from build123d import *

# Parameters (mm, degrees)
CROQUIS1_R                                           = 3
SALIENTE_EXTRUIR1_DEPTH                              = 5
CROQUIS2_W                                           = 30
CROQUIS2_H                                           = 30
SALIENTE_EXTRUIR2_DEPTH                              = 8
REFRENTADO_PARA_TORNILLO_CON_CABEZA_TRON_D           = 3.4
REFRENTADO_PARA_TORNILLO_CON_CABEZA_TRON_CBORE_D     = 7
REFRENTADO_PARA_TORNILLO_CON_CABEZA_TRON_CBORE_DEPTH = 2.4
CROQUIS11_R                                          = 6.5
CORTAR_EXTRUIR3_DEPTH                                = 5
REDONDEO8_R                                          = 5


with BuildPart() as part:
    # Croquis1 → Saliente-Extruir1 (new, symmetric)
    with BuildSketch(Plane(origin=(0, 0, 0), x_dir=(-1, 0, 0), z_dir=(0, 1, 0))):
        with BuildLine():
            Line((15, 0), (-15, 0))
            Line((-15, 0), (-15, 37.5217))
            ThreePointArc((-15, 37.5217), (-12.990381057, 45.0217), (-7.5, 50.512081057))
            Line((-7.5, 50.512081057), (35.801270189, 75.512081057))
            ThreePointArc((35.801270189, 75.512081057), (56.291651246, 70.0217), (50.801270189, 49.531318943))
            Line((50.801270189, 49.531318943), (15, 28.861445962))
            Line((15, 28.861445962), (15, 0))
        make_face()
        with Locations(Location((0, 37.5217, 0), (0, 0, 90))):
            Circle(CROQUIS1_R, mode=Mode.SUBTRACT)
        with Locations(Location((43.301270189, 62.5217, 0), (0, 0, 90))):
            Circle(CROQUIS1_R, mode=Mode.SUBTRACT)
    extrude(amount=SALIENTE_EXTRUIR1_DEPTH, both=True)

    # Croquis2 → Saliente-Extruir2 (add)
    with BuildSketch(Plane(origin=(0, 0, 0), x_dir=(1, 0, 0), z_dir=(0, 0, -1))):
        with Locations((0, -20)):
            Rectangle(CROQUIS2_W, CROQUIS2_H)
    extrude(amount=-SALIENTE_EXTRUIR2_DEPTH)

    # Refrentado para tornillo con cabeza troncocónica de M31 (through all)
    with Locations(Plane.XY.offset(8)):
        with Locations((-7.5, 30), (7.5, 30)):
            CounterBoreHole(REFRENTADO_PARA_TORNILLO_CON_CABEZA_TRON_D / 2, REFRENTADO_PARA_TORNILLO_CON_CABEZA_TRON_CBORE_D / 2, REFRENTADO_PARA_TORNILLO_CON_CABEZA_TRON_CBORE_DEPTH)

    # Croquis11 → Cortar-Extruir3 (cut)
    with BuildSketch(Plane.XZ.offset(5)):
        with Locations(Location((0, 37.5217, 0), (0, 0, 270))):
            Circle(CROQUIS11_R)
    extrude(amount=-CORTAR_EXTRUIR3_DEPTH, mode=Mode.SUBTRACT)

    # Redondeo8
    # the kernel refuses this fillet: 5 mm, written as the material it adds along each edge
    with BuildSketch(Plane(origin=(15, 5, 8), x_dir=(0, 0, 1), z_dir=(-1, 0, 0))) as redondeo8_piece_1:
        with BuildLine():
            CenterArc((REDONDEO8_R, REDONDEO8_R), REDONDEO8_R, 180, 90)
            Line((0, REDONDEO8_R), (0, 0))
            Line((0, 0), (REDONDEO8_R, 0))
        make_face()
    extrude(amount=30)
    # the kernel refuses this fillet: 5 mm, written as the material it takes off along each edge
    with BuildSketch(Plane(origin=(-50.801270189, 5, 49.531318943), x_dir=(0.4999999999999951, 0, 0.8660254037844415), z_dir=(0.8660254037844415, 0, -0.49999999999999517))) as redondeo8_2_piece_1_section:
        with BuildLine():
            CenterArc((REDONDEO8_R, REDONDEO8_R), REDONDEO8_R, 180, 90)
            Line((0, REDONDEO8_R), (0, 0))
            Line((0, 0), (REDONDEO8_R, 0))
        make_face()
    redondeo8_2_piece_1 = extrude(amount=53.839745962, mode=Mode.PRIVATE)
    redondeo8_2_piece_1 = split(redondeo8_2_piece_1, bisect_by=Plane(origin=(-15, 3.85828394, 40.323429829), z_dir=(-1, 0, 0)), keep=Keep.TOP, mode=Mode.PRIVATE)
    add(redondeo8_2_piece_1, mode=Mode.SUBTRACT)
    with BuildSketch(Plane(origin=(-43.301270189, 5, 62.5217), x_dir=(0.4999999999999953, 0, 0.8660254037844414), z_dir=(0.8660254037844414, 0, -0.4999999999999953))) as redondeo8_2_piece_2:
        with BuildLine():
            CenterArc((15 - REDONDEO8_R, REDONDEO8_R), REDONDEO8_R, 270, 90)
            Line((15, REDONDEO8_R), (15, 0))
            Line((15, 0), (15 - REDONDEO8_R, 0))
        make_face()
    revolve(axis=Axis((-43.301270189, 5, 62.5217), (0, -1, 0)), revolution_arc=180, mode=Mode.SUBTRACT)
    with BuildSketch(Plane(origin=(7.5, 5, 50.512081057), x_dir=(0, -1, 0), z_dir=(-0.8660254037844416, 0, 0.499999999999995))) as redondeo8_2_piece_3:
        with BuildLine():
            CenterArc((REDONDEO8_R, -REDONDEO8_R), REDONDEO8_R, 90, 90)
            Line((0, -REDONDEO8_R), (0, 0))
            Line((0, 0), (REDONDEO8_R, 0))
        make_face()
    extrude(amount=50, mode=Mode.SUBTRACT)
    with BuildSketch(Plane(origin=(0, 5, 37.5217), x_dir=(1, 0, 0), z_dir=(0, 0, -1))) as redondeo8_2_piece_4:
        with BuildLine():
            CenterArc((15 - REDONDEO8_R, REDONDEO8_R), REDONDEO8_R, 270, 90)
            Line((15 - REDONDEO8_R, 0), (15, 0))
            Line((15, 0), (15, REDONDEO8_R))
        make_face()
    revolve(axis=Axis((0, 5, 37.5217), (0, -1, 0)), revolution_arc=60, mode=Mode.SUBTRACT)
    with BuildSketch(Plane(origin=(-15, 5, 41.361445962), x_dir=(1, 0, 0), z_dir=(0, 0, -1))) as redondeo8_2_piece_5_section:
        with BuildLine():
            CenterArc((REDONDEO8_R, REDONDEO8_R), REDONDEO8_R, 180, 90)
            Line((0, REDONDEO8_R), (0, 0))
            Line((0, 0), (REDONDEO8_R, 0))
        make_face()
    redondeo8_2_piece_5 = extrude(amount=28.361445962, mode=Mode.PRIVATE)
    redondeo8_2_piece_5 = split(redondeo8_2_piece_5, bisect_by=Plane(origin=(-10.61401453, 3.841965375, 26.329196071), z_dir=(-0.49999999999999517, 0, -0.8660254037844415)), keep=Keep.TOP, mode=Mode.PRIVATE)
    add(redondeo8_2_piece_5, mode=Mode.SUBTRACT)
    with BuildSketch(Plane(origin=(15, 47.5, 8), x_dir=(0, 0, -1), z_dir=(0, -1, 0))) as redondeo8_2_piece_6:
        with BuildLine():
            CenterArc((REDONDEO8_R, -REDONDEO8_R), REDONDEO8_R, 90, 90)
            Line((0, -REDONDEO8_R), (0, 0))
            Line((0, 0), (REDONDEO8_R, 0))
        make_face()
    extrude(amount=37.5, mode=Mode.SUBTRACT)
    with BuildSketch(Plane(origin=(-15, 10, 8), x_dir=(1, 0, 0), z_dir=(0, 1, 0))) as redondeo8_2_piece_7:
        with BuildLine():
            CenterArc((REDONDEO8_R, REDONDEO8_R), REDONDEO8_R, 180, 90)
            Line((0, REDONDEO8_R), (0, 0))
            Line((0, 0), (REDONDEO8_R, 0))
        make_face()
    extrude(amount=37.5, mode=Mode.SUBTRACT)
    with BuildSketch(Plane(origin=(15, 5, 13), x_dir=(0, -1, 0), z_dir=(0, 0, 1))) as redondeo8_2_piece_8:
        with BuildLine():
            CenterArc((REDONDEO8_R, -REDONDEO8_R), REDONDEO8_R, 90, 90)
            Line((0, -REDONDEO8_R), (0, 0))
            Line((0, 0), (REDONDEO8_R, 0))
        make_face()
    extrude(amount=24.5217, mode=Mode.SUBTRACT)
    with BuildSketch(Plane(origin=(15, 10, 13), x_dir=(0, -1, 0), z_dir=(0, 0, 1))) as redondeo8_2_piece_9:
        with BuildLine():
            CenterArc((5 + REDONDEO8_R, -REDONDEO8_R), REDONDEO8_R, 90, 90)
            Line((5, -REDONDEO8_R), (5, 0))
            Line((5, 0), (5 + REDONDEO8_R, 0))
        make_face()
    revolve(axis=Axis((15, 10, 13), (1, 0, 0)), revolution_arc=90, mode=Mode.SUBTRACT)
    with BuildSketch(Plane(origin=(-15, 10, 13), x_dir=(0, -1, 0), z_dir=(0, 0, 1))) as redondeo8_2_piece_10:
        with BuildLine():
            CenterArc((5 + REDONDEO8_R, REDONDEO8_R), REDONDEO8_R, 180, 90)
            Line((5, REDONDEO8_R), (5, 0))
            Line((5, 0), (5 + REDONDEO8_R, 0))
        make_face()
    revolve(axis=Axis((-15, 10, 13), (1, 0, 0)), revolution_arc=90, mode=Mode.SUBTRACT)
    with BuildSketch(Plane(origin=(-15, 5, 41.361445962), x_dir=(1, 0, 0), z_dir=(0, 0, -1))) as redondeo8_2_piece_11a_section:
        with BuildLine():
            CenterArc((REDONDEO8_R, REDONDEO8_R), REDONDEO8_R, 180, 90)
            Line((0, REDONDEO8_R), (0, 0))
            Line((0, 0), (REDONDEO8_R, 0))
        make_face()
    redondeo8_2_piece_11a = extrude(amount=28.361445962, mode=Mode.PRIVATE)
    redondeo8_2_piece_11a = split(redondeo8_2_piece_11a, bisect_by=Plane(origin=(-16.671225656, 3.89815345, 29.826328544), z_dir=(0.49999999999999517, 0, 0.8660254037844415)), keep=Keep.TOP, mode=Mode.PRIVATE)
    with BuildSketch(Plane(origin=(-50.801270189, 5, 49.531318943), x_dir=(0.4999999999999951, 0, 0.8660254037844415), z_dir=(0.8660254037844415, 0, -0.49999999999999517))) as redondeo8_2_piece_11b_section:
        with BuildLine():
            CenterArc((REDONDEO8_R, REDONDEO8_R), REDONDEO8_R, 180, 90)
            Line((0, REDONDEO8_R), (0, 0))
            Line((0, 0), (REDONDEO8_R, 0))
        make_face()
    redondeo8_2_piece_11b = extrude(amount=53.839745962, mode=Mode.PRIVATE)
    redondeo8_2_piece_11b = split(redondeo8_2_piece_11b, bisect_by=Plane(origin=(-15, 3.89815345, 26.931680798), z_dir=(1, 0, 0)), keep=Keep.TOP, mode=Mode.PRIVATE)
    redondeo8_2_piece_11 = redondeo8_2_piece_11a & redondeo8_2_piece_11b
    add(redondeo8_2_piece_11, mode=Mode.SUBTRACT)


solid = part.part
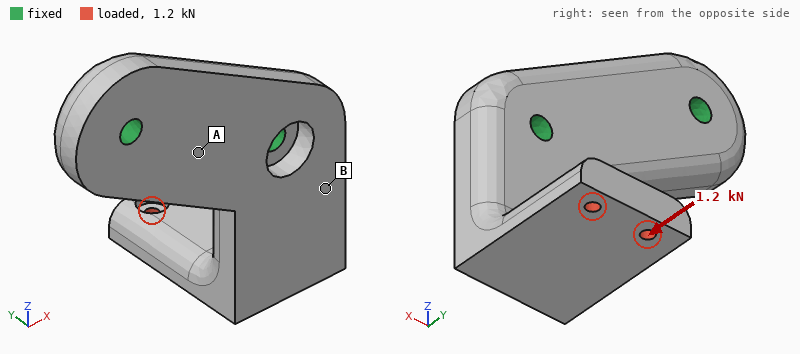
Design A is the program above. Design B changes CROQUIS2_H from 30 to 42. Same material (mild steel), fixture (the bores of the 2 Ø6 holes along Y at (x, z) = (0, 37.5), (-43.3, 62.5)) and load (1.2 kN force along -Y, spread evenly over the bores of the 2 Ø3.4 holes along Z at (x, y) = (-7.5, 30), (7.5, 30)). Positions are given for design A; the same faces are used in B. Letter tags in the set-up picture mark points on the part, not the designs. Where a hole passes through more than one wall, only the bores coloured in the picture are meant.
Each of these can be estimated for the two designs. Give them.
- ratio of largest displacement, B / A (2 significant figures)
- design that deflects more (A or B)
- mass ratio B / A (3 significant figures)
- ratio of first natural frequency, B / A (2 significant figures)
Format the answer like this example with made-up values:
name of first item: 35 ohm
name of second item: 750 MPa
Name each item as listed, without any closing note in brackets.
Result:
ratio of largest displacement, B / A: 1.1
design that deflects more: B
mass ratio B / A: 1.04
ratio of first natural frequency, B / A: 0.87
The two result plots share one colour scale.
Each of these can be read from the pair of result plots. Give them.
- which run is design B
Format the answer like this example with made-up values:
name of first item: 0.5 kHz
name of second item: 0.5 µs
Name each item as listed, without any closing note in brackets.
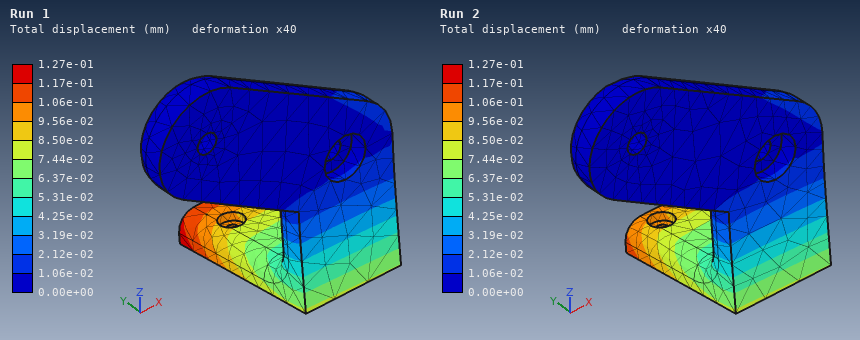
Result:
which run is design B: Run 1
